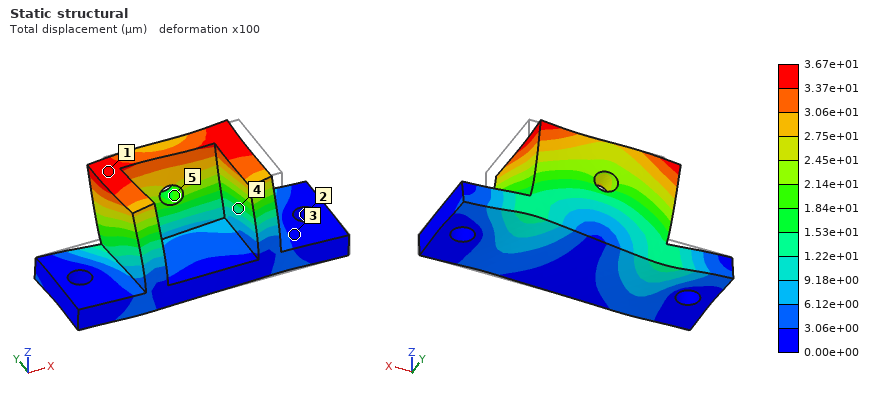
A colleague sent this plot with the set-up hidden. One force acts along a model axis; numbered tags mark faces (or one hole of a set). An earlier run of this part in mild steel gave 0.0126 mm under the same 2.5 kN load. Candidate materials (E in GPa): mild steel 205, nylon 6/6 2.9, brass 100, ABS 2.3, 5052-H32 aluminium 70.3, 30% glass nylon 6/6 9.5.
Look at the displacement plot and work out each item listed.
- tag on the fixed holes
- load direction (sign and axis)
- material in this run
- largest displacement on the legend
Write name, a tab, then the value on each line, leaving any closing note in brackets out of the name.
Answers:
tag on the fixed holes	2
load direction	-X
material in this run	5052-H32 aluminium
largest displacement on the legend	3.67e+01 µm
